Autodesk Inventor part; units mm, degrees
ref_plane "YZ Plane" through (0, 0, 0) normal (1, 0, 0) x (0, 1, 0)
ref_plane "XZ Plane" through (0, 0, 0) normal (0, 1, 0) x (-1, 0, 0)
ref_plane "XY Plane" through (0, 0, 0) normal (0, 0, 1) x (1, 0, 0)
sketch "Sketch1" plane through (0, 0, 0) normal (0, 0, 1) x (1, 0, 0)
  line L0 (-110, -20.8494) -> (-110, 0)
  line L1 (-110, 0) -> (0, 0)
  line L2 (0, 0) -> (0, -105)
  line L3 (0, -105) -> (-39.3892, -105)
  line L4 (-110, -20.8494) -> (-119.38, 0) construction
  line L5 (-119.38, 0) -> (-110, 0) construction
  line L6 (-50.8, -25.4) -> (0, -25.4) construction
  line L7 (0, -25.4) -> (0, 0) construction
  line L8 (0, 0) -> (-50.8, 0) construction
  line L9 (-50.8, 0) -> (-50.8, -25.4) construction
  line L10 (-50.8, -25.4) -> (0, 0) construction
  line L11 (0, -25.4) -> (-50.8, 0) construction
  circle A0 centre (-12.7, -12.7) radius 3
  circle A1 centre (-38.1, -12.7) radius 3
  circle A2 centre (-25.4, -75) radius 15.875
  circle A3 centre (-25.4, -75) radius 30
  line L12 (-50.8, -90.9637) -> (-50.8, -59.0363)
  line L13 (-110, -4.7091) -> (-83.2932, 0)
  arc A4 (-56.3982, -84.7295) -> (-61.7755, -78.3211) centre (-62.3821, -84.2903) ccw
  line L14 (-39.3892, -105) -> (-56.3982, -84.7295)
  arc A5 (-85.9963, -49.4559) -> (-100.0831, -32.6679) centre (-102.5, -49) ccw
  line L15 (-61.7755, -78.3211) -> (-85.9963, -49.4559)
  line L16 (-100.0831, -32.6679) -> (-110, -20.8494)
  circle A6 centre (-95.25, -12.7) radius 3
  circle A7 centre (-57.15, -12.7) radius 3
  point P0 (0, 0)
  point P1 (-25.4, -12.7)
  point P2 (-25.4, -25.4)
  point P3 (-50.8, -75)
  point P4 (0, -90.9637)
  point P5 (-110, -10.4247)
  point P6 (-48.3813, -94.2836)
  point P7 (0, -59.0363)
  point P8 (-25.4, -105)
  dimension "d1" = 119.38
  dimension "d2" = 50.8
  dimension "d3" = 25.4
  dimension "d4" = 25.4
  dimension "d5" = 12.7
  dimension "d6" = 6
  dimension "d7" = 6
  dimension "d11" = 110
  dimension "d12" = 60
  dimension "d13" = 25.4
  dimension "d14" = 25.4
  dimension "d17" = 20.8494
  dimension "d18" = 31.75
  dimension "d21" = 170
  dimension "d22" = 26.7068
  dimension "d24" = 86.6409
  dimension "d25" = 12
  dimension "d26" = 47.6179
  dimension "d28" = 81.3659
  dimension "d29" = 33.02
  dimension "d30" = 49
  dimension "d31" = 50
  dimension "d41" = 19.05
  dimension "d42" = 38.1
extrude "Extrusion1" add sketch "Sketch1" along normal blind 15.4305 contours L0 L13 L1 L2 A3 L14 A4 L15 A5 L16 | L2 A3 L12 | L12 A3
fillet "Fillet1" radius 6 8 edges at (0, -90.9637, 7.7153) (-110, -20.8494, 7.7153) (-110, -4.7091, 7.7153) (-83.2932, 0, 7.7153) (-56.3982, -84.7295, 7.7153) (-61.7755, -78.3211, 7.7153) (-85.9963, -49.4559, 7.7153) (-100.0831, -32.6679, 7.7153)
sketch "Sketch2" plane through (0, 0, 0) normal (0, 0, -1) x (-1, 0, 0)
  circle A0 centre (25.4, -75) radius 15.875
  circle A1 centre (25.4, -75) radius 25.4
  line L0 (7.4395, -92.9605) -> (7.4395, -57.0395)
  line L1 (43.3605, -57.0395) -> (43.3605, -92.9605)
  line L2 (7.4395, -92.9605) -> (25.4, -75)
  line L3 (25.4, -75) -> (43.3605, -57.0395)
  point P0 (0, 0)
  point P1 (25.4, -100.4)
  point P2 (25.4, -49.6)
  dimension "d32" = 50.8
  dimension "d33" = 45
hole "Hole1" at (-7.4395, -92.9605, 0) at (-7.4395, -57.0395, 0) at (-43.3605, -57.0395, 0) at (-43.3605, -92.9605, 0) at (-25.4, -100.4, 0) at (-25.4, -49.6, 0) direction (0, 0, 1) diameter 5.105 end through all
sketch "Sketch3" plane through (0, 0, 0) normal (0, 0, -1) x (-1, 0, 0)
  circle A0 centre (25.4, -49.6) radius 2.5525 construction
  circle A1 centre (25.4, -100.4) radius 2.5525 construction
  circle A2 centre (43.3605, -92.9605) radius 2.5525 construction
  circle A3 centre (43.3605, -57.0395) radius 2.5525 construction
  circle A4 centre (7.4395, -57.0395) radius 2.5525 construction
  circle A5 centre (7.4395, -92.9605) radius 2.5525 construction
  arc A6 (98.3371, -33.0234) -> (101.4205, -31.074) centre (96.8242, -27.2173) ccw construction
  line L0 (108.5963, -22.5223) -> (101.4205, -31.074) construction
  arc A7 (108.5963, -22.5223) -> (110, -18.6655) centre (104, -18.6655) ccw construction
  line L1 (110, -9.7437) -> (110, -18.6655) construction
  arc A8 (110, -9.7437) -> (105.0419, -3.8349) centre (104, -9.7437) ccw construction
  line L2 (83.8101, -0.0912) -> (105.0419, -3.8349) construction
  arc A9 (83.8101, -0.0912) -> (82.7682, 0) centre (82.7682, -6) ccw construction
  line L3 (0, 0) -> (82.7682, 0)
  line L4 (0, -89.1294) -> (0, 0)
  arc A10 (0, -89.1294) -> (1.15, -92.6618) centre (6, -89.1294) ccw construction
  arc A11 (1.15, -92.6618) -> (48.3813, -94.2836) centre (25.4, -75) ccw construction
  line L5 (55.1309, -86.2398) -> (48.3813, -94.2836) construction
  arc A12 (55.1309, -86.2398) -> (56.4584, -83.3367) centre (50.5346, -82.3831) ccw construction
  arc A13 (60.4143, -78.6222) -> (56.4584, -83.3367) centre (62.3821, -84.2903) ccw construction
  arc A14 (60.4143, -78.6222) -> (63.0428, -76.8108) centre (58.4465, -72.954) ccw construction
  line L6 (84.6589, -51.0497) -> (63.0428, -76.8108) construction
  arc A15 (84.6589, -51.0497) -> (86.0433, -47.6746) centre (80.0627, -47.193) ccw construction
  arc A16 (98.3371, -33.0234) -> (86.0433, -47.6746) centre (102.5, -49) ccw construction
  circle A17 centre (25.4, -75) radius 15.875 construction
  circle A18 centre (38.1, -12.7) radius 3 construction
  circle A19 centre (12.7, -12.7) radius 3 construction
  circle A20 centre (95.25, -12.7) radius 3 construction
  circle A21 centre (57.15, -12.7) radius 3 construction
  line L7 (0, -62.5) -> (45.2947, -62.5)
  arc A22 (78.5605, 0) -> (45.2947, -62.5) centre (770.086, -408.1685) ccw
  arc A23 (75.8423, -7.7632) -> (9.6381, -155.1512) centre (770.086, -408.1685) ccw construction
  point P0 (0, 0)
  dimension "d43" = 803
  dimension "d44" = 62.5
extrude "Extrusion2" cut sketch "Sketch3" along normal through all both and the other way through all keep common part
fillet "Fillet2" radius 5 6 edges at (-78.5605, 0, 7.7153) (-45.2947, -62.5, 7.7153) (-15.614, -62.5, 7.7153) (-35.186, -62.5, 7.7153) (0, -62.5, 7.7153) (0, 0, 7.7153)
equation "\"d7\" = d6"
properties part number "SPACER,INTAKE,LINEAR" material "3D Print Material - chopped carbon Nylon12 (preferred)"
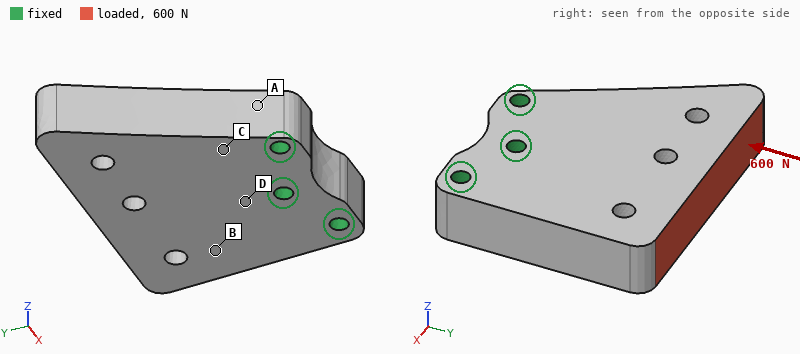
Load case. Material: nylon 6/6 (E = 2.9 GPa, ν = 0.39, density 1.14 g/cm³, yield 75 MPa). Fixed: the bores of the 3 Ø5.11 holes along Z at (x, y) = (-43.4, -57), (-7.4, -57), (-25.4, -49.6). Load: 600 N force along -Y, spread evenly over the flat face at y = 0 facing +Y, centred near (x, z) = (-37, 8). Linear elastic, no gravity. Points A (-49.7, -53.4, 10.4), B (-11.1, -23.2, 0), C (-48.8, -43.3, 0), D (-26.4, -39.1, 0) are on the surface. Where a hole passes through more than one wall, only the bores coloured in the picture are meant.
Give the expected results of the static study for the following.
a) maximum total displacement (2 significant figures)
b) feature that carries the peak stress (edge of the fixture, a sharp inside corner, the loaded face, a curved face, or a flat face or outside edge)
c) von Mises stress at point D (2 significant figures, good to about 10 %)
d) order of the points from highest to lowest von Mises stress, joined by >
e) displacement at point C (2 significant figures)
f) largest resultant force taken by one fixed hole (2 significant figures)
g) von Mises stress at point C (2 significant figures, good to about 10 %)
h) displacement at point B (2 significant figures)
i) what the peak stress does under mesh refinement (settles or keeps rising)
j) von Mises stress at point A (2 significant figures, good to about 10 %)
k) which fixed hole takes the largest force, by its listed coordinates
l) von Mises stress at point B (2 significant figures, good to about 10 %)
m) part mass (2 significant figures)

44 µm
edge of the fixture
0.84 MPa
A > C > D > B
11 µm
370 N
1.4 MPa
8.0 µm
keeps rising
1.8 MPa
(-43.4, -57)
0.40 MPa
64 g
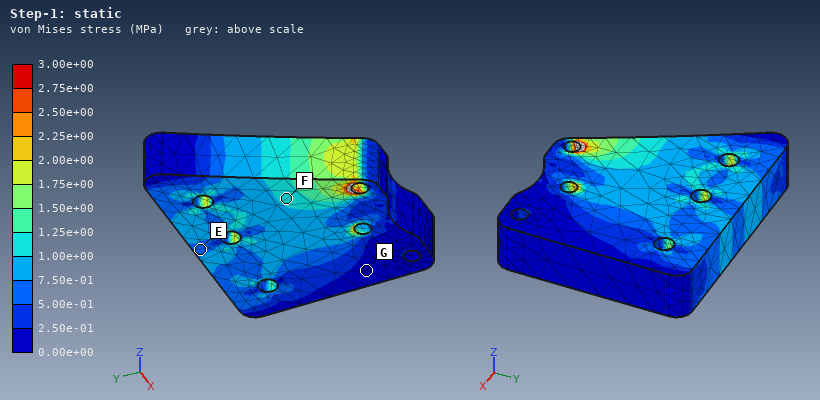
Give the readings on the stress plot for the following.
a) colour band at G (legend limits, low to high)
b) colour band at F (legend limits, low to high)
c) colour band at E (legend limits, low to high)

0.00e+00 to 2.50e-01 MPa
1.00e+00 to 1.25e+00 MPa
5.00e-01 to 7.50e-01 MPa
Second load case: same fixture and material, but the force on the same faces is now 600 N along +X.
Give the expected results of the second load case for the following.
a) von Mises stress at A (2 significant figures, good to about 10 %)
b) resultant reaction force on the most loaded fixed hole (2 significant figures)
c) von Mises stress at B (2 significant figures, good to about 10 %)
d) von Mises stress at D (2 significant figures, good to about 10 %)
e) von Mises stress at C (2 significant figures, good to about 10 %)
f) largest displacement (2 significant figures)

4.4 MPa
790 N
1.7 MPa
2.1 MPa
2.7 MPa
0.16 mm
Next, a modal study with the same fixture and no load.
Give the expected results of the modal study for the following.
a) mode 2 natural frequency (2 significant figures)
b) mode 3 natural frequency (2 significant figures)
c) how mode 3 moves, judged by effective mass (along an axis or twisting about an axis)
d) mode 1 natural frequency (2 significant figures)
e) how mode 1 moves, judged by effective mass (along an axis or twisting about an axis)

1900 Hz
2300 Hz
along X
1100 Hz
along Z
